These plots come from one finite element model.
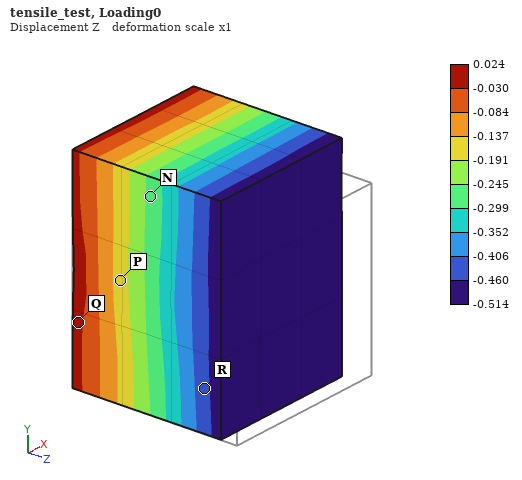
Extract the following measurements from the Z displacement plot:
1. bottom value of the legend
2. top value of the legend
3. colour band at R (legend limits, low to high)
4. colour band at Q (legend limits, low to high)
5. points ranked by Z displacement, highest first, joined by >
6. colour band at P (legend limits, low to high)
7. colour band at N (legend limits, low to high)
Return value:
-0.514
0.024
-0.460 to -0.406
-0.030 to 0.024
Q > P > N > R
-0.191 to -0.137
-0.299 to -0.245
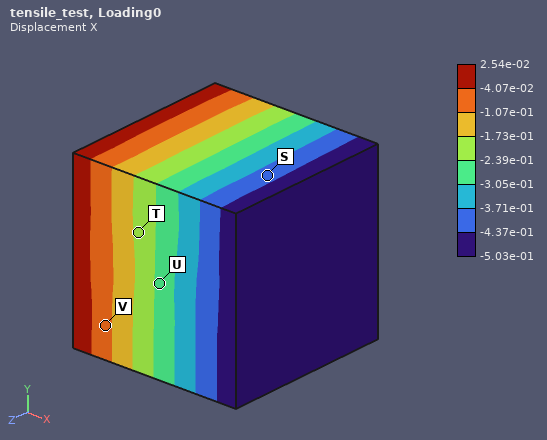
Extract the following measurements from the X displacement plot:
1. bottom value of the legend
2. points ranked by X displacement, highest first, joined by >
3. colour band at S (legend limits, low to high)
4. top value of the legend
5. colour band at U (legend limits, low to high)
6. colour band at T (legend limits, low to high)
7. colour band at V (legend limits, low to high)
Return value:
-5.03e-01
V > T > U > S
-4.37e-01 to -3.71e-01
2.54e-02
-3.05e-01 to -2.39e-01
-2.39e-01 to -1.73e-01
-1.07e-01 to -4.07e-02
